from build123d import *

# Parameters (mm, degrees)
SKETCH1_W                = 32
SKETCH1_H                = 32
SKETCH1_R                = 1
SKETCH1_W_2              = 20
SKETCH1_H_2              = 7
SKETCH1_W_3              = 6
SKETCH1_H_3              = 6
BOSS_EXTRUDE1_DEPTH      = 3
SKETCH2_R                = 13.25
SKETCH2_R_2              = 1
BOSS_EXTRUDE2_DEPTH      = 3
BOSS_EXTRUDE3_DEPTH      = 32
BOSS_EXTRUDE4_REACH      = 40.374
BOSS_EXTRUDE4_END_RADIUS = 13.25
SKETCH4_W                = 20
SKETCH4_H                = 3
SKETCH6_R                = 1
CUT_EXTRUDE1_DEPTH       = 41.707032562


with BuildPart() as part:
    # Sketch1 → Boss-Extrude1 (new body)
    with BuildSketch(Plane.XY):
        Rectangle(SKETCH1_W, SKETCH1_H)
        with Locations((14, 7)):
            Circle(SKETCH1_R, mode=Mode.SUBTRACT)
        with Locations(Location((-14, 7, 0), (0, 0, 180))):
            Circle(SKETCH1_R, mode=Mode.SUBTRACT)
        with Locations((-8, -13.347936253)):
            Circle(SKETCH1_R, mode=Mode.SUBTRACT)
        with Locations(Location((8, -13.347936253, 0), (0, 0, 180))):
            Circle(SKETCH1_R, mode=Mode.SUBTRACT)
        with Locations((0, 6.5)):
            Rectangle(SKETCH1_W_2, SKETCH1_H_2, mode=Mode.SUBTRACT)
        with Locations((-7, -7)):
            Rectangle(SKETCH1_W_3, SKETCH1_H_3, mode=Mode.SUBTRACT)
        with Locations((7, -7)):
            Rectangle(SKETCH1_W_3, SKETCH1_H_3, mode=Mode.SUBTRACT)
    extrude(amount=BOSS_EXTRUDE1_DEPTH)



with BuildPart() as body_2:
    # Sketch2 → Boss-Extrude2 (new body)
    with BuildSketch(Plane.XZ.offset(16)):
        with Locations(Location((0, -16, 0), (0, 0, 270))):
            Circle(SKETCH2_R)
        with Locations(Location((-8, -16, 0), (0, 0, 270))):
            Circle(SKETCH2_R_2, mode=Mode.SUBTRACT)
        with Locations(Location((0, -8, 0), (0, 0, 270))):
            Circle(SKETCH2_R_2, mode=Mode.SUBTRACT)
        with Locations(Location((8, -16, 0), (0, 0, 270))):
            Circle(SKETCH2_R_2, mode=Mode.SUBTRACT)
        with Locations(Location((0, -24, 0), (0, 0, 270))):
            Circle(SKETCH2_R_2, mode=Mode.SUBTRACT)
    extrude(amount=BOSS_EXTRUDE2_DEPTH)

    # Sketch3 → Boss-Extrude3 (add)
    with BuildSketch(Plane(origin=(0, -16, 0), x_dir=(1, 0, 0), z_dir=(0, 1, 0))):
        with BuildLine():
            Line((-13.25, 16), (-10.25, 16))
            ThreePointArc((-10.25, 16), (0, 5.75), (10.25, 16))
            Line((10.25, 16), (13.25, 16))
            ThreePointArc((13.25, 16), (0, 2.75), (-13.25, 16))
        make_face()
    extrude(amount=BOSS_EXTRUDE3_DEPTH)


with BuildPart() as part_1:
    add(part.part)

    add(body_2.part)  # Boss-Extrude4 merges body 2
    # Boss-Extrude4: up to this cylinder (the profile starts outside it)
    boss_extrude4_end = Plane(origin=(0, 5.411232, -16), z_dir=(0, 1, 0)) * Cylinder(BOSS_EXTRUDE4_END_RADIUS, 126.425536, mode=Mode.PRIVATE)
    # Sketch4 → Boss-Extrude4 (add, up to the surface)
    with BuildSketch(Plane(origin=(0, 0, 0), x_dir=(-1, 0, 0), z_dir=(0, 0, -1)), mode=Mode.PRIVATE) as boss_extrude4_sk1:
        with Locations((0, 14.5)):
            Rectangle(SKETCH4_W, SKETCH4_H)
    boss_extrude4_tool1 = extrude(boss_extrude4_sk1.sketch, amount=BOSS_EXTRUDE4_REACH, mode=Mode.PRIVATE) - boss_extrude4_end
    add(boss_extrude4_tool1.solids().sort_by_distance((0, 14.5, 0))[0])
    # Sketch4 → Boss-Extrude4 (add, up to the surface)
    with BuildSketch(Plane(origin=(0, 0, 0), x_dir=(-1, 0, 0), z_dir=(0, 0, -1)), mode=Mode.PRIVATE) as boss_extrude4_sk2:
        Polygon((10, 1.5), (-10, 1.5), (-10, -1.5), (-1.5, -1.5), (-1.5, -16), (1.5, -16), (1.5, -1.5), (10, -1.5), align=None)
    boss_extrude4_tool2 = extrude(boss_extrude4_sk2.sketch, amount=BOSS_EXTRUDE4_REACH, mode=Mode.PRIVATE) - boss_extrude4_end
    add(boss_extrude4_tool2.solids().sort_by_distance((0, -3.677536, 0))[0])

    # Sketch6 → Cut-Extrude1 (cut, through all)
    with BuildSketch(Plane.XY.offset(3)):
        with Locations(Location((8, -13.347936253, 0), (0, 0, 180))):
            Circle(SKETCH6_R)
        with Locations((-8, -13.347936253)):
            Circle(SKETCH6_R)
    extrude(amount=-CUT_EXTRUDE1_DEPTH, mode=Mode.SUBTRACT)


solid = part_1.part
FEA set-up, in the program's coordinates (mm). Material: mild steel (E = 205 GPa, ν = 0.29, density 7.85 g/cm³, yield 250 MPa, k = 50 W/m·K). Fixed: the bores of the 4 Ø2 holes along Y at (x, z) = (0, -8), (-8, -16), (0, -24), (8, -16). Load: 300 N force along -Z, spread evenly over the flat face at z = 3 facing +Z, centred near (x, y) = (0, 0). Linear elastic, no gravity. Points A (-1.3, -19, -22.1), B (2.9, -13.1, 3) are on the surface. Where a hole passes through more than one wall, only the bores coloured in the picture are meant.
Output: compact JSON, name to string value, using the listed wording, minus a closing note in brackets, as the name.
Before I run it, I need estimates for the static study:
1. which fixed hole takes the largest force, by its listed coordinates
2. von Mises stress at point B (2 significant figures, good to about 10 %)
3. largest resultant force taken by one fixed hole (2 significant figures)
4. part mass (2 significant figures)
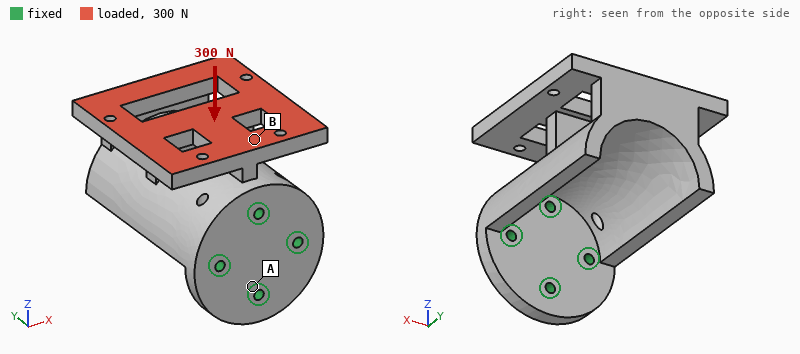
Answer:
{"which fixed hole takes the largest force, by its listed coordinates": "(0, -8)", "von Mises stress at point B": "12 MPa", "largest resultant force taken by one fixed hole": "510 N", "part mass": "64 g"}
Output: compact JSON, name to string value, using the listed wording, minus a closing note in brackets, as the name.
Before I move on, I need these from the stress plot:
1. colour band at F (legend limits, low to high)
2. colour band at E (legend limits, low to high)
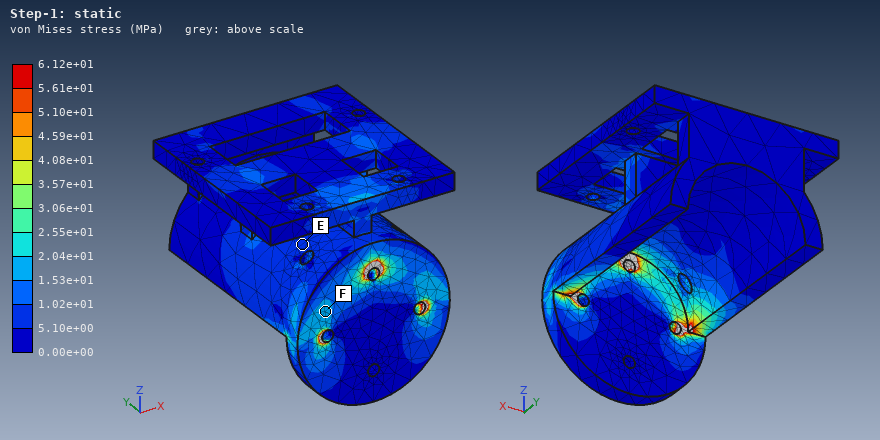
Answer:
{"colour band at F": "1.53e+01 to 2.04e+01 MPa", "colour band at E": "5.10e+00 to 1.02e+01 MPa"}
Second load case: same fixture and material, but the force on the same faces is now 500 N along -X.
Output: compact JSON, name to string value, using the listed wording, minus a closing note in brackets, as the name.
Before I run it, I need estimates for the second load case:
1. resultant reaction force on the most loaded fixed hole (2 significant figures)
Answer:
{"resultant reaction force on the most loaded fixed hole": "500 N"}
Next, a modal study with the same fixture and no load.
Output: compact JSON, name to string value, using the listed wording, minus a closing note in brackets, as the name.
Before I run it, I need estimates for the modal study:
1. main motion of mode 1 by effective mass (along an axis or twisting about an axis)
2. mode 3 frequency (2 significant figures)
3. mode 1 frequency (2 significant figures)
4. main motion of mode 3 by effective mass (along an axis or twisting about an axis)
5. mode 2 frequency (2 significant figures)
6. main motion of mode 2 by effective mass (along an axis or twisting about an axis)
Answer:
{"main motion of mode 1 by effective mass": "along Z", "mode 3 frequency": "6300 Hz", "mode 1 frequency": "3400 Hz", "main motion of mode 3 by effective mass": "along X", "mode 2 frequency": "3600 Hz", "main motion of mode 2 by effective mass": "along X"}
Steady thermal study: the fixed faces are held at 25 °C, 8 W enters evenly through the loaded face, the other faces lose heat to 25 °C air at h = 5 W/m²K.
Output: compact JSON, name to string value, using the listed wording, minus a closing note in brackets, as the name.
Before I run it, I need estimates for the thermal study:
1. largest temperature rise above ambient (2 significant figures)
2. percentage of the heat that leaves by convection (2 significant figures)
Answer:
{"largest temperature rise above ambient": "35 K", "percentage of the heat that leaves by convection": "7.1 %"}
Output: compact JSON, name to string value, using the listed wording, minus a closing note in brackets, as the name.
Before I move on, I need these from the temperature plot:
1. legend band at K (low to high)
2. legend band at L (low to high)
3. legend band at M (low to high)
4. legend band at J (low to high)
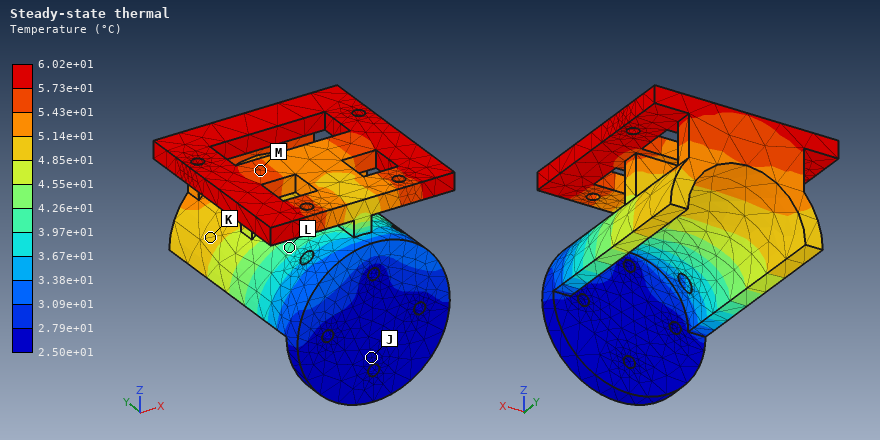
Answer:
{"legend band at K": "4.85e+01 to 5.14e+01 °C", "legend band at L": "3.97e+01 to 4.26e+01 °C", "legend band at M": "5.43e+01 to 5.73e+01 °C", "legend band at J": "2.50e+01 to 2.79e+01 °C"}
